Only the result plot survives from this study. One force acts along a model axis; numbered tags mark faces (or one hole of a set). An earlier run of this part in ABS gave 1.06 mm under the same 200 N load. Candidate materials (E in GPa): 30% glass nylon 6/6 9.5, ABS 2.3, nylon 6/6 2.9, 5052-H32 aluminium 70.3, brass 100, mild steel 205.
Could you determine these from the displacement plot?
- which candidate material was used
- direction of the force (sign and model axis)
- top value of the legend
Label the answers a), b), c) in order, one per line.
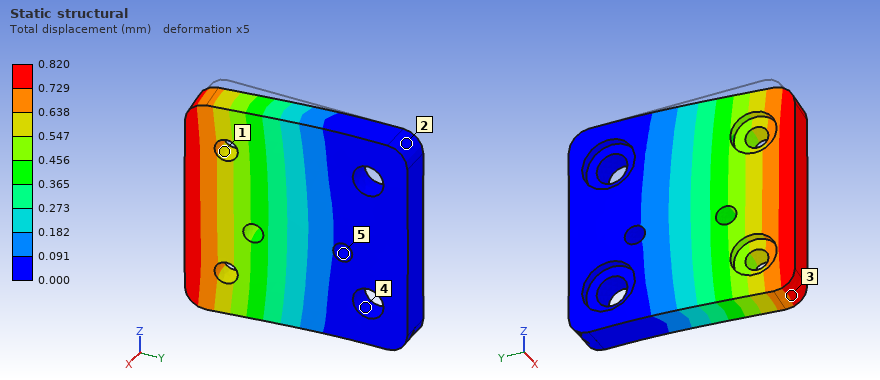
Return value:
a) nylon 6/6
b) +X
c) 0.820 mm
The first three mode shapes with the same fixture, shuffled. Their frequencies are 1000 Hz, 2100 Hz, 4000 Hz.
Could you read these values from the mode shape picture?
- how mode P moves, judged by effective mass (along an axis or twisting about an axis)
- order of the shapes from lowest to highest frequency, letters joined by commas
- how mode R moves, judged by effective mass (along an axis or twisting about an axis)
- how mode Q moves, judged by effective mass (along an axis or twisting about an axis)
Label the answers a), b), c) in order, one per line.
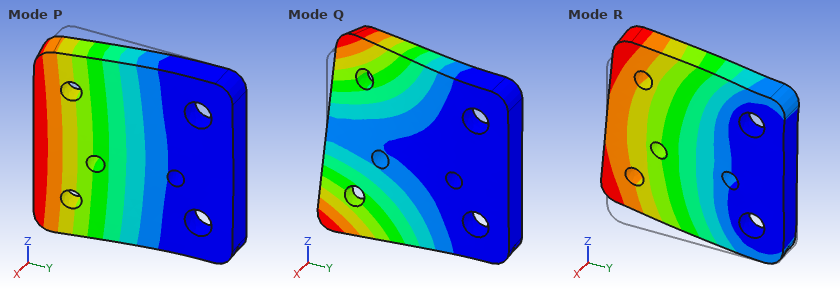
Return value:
a) along X
b) P, Q, R
c) along Z
d) twisting about Y
